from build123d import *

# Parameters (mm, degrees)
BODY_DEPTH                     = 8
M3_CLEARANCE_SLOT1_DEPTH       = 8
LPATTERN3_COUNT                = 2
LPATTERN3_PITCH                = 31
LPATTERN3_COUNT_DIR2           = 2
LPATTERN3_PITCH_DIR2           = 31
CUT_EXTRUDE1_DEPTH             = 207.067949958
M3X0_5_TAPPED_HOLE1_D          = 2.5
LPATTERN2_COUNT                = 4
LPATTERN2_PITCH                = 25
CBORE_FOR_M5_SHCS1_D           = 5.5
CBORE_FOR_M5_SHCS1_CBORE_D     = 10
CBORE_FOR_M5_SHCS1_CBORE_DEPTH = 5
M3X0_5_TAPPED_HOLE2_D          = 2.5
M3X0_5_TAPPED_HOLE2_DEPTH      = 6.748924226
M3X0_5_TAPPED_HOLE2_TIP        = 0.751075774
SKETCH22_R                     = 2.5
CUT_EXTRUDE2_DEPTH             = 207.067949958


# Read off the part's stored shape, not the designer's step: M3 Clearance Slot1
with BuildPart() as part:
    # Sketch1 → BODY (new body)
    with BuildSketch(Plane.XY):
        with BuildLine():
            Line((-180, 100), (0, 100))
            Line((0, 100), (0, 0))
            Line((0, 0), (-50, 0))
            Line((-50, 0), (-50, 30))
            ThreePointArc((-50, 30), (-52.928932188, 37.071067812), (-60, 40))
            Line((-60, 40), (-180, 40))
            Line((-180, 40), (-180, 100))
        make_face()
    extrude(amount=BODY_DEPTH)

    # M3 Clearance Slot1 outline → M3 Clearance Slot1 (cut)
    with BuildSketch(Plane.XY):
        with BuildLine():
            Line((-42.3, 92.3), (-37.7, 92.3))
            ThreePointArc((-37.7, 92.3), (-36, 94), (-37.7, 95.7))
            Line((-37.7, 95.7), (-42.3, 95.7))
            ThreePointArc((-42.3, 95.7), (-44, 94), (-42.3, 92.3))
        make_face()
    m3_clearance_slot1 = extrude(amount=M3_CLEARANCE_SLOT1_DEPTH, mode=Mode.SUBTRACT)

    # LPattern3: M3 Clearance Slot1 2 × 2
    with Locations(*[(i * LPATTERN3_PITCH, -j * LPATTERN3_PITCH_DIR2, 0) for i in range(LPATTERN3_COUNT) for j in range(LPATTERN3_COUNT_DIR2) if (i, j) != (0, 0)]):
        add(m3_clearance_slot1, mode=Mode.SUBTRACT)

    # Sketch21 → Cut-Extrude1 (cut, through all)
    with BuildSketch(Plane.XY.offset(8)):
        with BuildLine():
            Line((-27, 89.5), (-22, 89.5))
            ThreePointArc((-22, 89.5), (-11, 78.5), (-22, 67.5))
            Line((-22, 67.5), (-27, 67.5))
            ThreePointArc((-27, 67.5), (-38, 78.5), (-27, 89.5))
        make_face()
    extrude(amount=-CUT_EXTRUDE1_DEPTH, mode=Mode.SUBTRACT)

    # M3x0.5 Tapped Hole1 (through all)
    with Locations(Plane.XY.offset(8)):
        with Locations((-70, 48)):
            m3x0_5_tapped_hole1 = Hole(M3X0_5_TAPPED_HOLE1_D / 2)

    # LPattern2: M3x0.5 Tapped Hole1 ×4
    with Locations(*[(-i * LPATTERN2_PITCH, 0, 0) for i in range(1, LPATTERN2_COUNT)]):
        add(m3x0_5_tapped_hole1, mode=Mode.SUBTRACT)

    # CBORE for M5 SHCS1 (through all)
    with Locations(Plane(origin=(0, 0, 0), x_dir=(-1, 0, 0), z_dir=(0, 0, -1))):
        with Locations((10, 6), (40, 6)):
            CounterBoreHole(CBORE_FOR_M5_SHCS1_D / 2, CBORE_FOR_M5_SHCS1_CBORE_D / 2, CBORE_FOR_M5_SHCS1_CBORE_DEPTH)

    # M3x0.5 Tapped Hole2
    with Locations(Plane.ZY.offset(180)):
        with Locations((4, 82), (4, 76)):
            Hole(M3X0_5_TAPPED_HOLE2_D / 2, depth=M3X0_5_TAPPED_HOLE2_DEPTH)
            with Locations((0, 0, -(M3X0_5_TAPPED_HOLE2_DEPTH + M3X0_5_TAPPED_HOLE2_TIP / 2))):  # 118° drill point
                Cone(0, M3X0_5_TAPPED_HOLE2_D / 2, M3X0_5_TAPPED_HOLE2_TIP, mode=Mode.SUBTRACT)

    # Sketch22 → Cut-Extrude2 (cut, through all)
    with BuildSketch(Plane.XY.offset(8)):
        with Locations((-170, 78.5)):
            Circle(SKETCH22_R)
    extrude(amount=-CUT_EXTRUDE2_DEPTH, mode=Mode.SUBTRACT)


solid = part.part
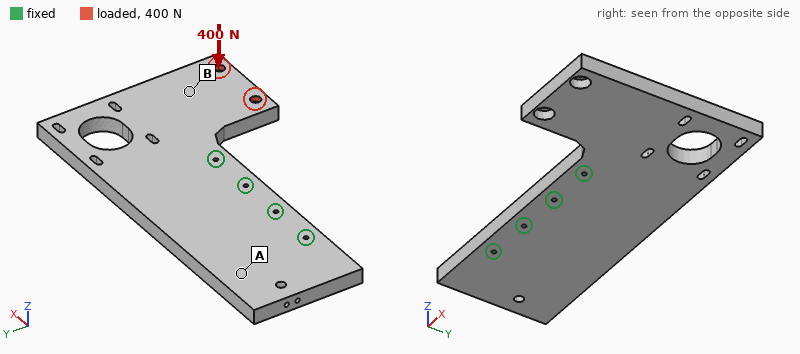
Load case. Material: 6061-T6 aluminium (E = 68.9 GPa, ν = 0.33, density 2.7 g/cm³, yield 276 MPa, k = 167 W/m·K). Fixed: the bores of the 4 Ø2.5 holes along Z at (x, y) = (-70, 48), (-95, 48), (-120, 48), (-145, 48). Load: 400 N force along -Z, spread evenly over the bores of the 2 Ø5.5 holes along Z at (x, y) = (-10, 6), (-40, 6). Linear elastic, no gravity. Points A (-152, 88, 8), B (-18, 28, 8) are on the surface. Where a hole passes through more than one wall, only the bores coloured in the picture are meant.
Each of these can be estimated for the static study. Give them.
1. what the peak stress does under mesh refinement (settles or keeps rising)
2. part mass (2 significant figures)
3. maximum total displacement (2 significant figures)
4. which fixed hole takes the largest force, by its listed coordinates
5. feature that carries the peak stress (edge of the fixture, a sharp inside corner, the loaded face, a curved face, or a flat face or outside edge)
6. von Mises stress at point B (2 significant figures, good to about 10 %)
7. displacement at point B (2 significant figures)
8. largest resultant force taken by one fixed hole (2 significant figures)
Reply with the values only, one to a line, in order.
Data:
keeps rising
260 g
0.55 mm
(-70, 48)
edge of the fixture
15 MPa
0.28 mm
800 N
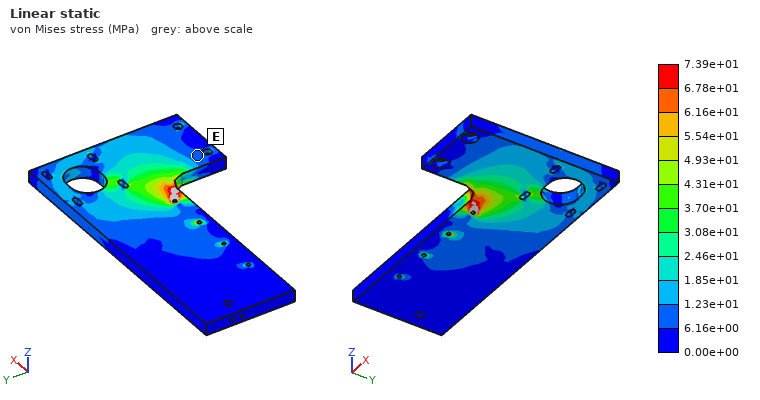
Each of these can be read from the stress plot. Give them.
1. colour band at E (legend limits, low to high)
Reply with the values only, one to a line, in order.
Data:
6.16e+00 to 1.23e+01 MPa
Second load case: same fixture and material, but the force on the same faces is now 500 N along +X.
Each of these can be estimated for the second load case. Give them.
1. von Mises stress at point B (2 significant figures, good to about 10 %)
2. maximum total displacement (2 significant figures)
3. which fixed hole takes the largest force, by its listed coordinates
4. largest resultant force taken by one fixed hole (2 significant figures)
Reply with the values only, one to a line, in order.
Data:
4.1 MPa
42 µm
(-70, 48)
780 N
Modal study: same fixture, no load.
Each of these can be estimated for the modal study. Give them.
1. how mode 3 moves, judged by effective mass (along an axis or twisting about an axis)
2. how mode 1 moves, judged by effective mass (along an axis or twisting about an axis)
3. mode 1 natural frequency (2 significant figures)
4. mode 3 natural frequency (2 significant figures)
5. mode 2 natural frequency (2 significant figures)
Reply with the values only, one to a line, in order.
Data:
along Z
along Z
840 Hz
1900 Hz
1100 Hz
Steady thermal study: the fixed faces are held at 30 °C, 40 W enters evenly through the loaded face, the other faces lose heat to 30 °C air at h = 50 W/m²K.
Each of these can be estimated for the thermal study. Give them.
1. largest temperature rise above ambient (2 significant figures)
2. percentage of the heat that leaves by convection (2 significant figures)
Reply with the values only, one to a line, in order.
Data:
49 K
41 %
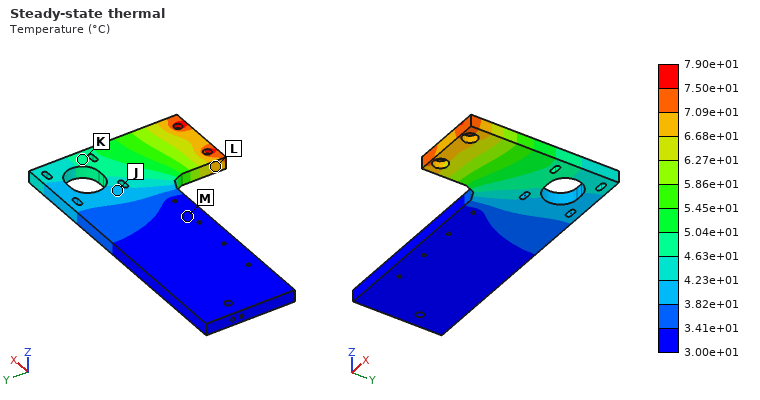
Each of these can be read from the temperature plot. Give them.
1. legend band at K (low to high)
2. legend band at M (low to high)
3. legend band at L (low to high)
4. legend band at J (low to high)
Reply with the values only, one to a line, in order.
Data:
4.63e+01 to 5.04e+01 °C
3.00e+01 to 3.41e+01 °C
6.68e+01 to 7.09e+01 °C
3.82e+01 to 4.23e+01 °C
